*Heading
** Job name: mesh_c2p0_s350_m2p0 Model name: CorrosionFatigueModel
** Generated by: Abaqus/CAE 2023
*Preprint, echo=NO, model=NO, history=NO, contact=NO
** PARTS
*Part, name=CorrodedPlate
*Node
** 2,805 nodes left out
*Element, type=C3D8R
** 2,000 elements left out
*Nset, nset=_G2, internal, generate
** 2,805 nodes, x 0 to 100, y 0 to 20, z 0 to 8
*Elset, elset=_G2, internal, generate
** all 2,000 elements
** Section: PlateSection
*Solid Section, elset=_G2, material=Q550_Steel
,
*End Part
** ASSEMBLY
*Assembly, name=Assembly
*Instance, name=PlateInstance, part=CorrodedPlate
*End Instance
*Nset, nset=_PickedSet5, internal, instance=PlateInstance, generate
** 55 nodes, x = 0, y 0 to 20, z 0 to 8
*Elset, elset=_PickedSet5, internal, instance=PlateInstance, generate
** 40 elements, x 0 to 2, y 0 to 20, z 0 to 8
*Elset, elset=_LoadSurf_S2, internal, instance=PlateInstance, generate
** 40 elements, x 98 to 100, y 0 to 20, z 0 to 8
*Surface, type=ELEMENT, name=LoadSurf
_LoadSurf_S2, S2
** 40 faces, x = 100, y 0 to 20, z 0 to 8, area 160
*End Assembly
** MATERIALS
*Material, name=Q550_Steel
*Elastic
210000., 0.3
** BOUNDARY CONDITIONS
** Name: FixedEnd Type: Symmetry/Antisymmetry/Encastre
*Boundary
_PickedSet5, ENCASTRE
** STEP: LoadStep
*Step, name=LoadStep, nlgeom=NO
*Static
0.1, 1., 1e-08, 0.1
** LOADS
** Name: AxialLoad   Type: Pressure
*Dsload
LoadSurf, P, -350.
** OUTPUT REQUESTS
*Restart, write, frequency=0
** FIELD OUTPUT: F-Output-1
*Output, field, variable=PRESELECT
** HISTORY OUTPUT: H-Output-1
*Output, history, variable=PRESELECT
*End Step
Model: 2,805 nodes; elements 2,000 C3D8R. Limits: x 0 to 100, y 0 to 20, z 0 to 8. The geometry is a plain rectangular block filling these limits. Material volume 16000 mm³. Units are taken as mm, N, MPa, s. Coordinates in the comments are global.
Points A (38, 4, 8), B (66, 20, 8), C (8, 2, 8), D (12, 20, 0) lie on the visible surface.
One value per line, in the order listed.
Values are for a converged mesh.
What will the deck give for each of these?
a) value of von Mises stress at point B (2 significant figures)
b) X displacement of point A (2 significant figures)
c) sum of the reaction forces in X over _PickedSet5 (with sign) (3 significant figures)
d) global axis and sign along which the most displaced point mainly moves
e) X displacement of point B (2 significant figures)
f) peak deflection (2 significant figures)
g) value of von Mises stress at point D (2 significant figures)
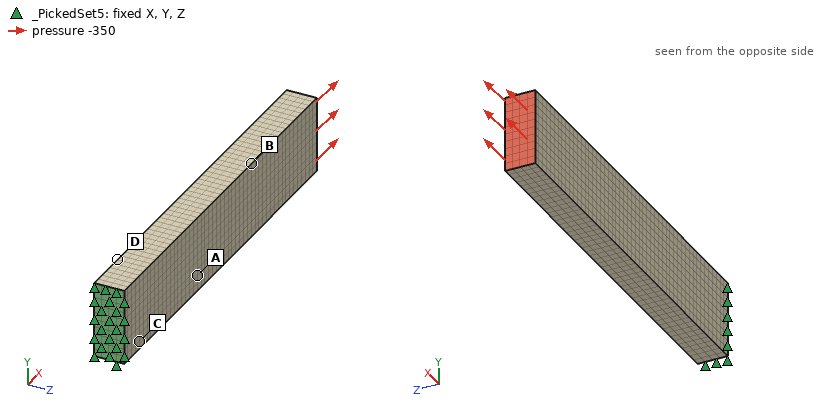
350 MPa
0.063 mm
-56000 N
+X
0.11 mm
0.17 mm
340 MPa
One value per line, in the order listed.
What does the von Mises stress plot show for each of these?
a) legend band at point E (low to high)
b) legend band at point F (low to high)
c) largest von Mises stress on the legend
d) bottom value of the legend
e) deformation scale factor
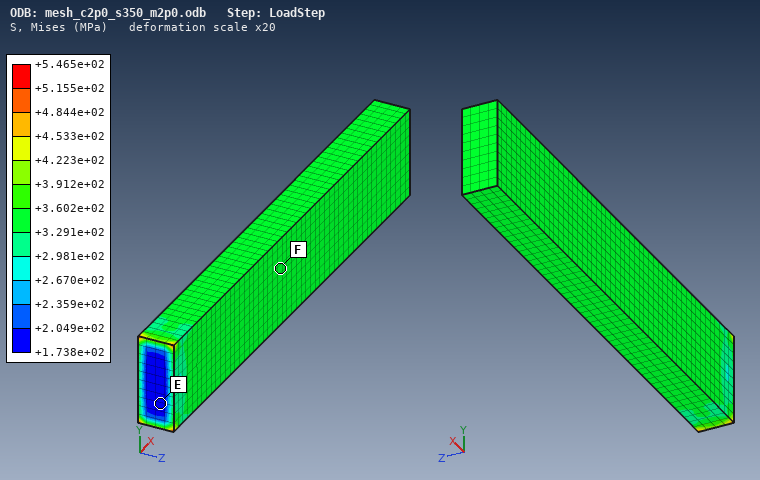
+1.738e+02 to +2.049e+02 MPa
+3.291e+02 to +3.602e+02 MPa
+5.465e+02 MPa
+1.738e+02 MPa
20
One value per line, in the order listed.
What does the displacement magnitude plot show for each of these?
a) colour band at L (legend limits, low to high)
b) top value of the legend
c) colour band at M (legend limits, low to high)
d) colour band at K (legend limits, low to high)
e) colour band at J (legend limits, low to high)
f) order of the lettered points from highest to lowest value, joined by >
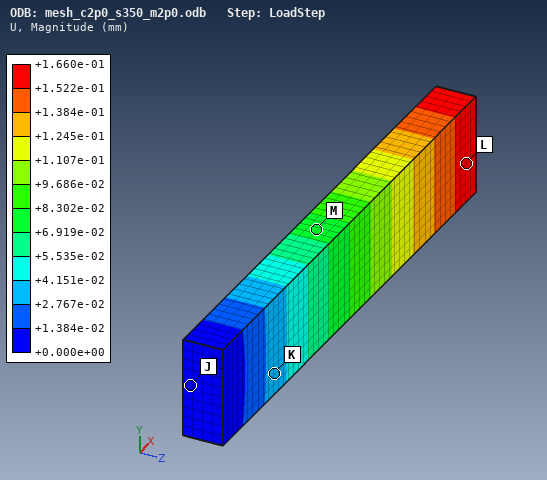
+1.522e-01 to +1.660e-01 mm
+1.660e-01 mm
+6.919e-02 to +8.302e-02 mm
+2.767e-02 to +4.151e-02 mm
+0.000e+00 to +1.384e-02 mm
L > M > K > J
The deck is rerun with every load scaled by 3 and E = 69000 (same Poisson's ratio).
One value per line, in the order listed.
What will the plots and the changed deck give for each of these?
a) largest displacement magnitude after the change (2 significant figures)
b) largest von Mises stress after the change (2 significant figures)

1.5 mm
1600 MPa
